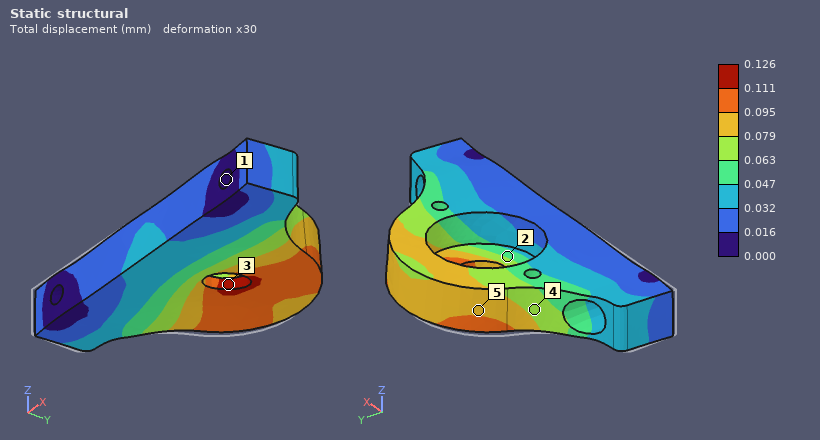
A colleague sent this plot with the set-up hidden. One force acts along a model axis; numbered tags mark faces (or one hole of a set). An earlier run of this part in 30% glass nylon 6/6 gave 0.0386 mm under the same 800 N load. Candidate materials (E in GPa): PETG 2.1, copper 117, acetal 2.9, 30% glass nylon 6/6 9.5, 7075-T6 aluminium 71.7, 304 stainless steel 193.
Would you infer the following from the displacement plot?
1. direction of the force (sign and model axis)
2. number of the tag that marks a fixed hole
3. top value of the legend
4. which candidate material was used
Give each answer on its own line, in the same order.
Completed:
+X
1
0.126 mm
acetal
